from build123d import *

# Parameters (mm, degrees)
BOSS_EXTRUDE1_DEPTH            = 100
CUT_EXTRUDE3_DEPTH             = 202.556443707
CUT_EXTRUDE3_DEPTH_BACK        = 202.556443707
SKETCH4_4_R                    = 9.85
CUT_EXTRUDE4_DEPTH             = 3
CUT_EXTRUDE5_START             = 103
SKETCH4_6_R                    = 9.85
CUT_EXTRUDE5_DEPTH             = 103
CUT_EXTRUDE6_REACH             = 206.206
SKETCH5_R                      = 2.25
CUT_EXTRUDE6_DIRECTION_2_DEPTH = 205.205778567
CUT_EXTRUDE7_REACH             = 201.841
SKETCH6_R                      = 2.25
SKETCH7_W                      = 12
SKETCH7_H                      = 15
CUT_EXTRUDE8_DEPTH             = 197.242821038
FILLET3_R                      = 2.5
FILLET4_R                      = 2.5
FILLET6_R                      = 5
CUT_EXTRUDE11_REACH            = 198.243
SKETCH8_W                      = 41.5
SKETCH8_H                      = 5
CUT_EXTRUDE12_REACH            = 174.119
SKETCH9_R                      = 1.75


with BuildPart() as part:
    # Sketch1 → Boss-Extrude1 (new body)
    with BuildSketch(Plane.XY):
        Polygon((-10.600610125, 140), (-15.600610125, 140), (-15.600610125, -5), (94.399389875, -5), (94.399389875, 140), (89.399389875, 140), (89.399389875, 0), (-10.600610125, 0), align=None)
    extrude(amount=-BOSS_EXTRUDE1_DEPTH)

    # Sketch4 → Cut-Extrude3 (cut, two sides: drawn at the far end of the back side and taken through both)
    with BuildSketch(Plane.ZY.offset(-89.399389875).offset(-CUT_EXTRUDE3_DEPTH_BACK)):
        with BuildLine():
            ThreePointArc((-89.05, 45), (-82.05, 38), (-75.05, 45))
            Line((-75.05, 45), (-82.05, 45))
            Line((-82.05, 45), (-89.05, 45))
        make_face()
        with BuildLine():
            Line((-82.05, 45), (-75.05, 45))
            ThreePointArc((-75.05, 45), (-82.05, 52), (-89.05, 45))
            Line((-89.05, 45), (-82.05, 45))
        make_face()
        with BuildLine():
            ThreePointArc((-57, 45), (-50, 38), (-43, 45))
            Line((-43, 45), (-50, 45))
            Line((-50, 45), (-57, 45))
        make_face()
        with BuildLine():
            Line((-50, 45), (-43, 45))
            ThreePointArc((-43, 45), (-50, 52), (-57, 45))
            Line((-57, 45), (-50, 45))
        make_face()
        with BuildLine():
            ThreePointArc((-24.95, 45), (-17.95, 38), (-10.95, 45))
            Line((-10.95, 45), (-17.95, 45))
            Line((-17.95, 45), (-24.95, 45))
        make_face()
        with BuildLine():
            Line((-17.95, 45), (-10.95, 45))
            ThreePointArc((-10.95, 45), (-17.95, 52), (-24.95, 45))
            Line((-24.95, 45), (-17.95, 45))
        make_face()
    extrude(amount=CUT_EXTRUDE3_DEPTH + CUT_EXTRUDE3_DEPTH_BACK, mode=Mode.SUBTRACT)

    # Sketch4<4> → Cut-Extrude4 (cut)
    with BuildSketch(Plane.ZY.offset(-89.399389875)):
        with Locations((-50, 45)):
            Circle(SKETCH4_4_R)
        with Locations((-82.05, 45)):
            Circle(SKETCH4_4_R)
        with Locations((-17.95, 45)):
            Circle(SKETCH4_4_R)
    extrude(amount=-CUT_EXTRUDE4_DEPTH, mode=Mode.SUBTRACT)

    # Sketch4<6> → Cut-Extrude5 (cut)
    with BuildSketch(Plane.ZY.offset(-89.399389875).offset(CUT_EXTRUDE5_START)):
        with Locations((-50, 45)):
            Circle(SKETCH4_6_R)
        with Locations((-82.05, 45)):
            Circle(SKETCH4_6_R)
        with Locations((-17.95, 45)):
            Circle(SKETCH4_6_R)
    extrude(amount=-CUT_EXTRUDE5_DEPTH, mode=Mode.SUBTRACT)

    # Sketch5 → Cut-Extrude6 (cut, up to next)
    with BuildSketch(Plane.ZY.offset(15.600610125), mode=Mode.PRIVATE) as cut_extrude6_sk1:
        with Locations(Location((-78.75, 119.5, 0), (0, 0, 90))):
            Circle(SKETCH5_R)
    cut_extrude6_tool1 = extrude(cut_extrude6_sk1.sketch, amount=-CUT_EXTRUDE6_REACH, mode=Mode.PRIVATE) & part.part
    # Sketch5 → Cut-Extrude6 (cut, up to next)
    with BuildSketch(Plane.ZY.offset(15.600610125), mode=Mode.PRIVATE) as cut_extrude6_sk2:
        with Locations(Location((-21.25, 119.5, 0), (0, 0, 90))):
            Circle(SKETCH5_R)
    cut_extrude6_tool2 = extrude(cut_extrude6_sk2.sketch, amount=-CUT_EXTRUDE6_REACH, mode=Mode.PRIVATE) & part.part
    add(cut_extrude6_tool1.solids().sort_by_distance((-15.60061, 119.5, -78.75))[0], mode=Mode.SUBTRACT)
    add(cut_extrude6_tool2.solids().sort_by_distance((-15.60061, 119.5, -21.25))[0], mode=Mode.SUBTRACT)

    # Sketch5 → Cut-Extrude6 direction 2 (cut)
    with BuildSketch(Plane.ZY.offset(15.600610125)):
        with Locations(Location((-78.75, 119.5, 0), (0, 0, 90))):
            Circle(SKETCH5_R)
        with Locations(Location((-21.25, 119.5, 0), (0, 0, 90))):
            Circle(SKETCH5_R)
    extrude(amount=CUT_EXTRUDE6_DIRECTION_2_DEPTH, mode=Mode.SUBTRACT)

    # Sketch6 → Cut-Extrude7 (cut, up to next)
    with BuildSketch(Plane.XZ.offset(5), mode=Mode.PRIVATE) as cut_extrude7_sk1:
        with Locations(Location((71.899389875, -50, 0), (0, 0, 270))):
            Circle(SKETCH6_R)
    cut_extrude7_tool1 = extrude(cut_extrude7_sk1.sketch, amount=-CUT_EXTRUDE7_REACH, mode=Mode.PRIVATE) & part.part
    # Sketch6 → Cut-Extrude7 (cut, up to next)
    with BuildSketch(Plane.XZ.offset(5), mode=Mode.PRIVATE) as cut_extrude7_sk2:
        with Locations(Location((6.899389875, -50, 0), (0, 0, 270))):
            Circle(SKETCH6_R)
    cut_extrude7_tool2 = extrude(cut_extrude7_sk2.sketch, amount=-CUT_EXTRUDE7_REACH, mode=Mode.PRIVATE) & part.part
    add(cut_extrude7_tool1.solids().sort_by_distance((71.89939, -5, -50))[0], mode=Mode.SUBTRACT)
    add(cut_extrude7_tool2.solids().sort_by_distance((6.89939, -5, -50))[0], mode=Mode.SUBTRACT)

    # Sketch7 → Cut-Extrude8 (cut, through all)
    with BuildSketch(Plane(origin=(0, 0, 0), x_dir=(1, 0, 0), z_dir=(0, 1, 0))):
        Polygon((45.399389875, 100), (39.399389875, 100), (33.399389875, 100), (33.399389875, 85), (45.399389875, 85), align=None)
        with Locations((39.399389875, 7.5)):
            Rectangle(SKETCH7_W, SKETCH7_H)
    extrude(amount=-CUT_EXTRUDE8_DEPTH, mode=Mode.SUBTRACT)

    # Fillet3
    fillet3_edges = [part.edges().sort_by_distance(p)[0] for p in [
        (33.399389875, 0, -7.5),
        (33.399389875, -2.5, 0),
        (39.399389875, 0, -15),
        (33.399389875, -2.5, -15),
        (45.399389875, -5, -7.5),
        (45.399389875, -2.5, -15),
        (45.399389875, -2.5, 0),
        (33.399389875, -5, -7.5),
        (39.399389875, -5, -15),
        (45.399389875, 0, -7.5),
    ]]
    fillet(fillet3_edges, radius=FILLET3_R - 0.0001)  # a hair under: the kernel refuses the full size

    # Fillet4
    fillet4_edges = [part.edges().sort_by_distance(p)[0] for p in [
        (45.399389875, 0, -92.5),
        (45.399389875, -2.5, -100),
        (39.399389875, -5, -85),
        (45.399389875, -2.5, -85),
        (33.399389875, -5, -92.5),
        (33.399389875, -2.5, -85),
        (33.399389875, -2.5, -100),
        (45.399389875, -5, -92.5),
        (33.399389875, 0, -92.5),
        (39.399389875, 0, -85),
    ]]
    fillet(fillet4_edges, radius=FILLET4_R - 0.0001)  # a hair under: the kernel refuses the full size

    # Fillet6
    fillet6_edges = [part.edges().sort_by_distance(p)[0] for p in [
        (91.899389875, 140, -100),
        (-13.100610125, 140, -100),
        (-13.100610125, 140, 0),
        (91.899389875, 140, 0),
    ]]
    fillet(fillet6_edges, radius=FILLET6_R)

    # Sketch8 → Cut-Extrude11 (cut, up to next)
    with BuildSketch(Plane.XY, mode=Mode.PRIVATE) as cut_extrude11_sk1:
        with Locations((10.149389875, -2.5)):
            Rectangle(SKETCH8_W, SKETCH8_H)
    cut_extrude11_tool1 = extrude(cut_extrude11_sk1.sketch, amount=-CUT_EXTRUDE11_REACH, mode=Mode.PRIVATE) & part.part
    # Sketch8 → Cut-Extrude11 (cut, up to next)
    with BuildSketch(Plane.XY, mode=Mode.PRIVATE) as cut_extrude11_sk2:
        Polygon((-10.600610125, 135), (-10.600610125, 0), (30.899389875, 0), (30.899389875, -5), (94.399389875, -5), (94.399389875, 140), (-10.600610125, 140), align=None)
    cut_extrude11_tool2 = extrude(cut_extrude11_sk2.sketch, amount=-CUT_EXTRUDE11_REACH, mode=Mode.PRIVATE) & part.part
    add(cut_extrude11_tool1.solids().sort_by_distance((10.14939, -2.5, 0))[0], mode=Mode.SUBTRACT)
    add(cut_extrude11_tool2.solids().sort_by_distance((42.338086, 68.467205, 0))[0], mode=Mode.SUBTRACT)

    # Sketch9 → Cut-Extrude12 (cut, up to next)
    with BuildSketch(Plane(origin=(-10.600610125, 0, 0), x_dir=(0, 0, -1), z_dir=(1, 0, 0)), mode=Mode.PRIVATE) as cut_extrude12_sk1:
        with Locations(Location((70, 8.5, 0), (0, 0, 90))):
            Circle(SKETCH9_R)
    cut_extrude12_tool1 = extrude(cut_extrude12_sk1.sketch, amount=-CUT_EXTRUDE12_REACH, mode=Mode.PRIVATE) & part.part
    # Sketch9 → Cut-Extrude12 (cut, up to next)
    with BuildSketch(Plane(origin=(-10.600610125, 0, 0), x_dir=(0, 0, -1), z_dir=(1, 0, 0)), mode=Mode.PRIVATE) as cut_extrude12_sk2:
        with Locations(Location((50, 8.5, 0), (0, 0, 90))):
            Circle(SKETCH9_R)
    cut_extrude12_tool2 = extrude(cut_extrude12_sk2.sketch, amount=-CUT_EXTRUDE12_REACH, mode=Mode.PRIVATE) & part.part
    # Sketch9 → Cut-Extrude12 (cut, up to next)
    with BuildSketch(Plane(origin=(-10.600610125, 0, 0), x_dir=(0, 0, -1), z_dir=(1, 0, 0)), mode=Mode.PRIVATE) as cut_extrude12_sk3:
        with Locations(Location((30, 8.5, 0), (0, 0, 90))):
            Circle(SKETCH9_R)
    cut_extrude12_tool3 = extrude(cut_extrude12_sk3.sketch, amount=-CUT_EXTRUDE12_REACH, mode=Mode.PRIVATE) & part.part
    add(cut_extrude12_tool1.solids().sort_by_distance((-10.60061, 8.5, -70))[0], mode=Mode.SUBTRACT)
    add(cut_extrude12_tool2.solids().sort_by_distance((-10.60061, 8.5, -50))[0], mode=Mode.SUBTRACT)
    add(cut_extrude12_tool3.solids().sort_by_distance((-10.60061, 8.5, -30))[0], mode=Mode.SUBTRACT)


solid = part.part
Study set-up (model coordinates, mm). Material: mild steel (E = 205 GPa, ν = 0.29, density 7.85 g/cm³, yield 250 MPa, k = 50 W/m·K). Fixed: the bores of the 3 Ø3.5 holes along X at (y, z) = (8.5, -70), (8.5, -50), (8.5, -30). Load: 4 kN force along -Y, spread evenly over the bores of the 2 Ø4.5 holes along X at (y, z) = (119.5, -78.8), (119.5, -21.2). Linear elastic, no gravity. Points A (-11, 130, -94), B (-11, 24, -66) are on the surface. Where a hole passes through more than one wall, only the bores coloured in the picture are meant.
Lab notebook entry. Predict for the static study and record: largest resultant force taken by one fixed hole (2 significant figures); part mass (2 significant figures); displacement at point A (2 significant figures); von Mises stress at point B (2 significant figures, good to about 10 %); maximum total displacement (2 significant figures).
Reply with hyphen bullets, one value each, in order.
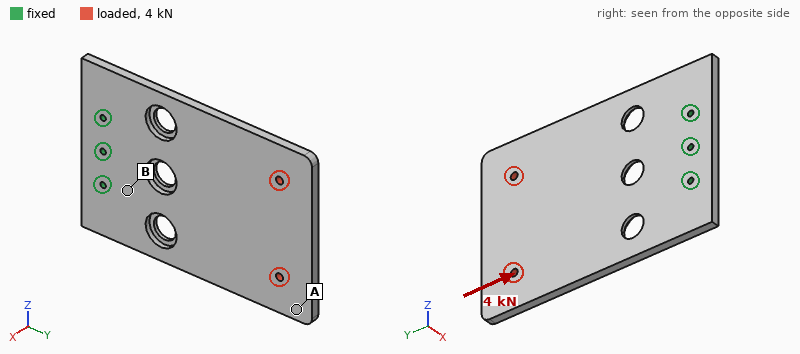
- 1.6 kN
- 540 g
- 17 µm
- 15 MPa
- 19 µm
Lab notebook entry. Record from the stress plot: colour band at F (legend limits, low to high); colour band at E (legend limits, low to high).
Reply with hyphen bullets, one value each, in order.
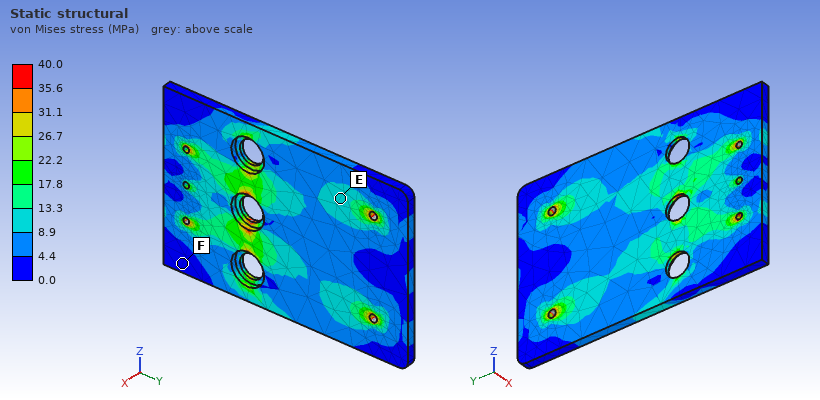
- 0.0 to 4.4 MPa
- 8.9 to 13.3 MPa
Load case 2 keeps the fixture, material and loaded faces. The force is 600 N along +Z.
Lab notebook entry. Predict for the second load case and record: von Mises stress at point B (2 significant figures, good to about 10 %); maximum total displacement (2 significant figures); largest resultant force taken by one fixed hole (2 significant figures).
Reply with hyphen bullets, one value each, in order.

- 10 MPa
- 19 µm
- 1.6 kN
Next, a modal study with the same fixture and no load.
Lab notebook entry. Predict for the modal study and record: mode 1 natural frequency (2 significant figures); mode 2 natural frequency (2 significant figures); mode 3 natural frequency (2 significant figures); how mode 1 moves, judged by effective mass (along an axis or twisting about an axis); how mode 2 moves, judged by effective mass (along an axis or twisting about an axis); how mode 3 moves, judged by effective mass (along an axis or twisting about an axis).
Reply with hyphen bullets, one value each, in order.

- 210 Hz
- 630 Hz
- 1400 Hz
- along X
- twisting about Y
- along X
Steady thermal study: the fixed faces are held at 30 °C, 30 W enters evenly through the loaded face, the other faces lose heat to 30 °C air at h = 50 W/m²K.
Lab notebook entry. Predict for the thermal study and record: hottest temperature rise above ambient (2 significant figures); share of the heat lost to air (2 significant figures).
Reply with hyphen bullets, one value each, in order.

- 55 K
- 90 %
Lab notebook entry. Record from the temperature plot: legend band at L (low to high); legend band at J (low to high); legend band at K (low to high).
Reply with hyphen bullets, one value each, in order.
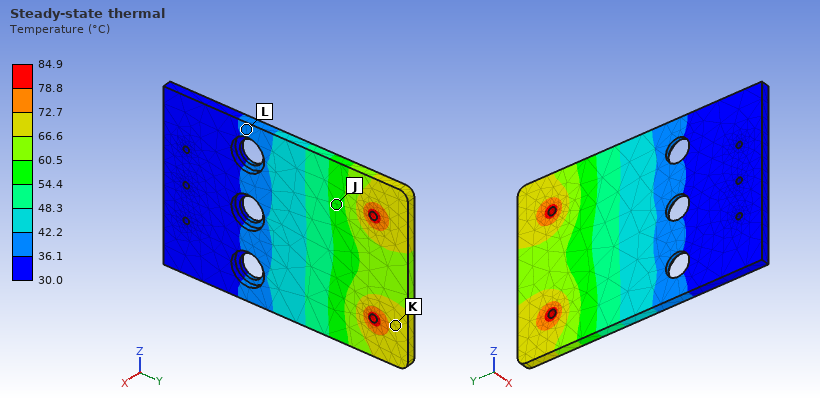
- 36.1 to 42.2 °C
- 54.4 to 60.5 °C
- 66.6 to 72.7 °C
